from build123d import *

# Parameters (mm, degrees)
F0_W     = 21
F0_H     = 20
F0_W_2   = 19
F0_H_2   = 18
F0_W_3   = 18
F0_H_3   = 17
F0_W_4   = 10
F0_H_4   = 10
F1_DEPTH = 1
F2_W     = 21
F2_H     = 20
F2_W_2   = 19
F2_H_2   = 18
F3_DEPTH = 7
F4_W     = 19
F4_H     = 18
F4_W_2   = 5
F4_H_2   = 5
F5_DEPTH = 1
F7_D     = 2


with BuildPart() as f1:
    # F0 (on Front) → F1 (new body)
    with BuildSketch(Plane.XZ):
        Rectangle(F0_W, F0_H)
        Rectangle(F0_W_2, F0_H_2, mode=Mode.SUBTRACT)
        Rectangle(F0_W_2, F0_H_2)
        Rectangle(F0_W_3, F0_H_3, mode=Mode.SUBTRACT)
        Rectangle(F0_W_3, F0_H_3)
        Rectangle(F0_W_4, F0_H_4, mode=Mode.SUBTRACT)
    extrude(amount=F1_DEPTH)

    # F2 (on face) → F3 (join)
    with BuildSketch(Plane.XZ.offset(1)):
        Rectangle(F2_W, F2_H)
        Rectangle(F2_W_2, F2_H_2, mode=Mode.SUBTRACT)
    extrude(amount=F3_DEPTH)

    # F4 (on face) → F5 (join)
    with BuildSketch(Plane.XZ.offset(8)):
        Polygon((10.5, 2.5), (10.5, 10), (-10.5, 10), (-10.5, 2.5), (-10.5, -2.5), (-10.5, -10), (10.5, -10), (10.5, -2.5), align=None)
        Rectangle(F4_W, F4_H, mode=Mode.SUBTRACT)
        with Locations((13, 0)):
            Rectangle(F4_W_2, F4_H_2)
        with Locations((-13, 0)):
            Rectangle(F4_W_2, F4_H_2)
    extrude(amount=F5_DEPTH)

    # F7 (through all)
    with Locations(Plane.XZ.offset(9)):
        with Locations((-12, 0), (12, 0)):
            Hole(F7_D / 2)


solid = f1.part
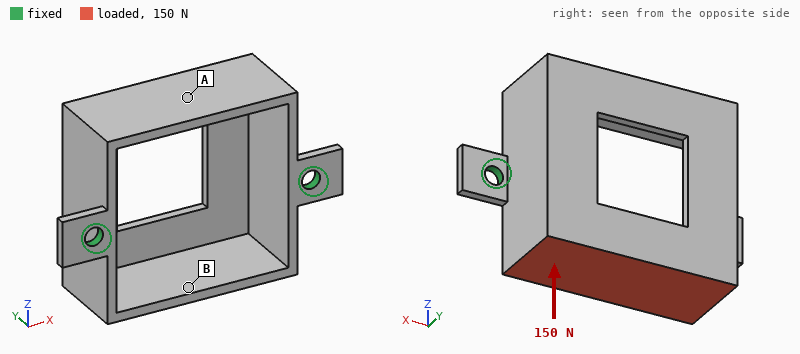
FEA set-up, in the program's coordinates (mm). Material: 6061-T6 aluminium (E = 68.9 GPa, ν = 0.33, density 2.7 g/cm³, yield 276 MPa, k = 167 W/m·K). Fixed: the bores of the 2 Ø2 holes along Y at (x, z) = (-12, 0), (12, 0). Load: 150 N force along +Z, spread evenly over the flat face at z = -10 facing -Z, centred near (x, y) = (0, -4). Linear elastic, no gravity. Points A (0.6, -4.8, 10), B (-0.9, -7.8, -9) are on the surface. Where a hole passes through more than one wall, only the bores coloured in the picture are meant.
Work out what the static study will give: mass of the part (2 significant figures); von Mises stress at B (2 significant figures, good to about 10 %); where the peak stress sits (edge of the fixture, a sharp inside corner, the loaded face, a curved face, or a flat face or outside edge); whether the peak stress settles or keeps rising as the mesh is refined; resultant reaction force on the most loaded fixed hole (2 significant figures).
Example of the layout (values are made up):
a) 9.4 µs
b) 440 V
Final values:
a) 2.7 g
b) 50 MPa
c) edge of the fixture
d) keeps rising
e) 75 N
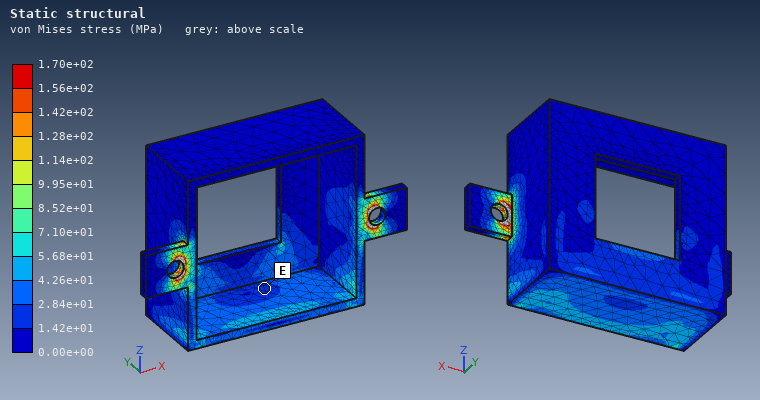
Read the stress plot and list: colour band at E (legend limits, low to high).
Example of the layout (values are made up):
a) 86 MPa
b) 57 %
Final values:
a) 1.42e+01 to 2.84e+01 MPa
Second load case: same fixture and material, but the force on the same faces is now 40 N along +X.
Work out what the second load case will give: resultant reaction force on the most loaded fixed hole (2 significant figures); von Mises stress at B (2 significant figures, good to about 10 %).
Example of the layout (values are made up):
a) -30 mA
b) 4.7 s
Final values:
a) 25 N
b) 11 MPa
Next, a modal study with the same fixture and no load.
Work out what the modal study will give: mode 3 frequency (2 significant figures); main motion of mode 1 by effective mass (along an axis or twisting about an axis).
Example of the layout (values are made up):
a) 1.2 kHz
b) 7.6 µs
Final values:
a) 5900 Hz
b) along Z
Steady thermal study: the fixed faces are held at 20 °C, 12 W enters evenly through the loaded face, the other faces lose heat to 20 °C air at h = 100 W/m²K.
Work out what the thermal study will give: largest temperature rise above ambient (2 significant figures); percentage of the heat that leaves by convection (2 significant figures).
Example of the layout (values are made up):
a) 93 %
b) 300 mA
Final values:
a) 45 K
b) 31 %
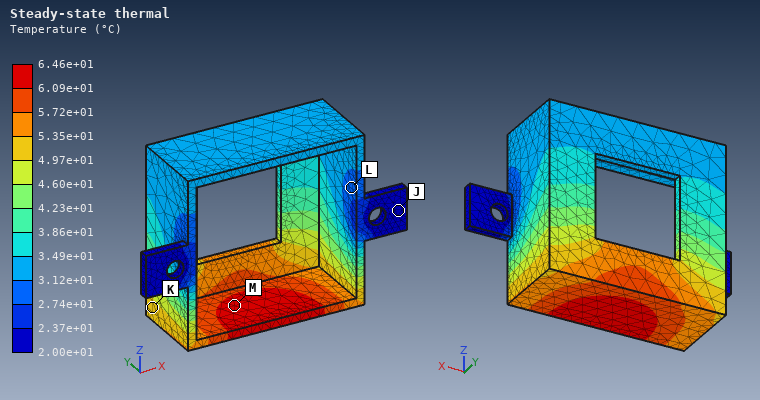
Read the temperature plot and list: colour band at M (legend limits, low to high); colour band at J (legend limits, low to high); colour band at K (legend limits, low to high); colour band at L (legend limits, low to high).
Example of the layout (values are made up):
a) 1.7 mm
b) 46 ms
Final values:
a) 6.09e+01 to 6.46e+01 °C
b) 2.00e+01 to 2.37e+01 °C
c) 4.97e+01 to 5.35e+01 °C
d) 2.74e+01 to 3.12e+01 °C
